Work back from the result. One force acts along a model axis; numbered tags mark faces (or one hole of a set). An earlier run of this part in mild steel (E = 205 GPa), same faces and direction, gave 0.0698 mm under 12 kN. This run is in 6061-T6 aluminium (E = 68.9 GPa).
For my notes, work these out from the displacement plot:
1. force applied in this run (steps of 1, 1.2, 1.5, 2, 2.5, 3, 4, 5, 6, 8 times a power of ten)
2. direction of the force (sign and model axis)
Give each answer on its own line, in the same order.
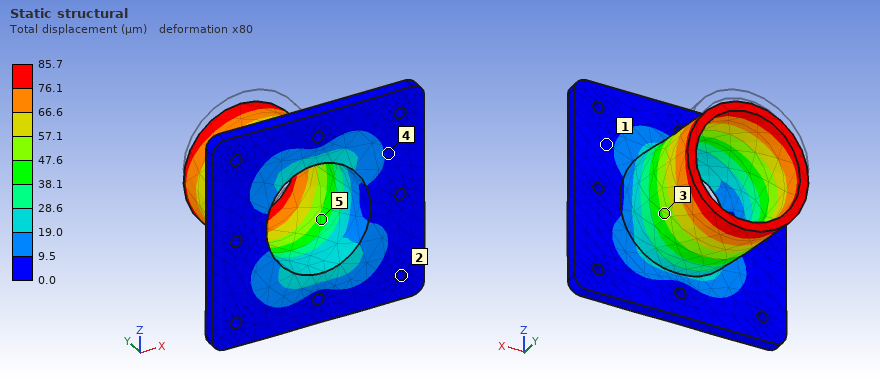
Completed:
5 kN
-Z
